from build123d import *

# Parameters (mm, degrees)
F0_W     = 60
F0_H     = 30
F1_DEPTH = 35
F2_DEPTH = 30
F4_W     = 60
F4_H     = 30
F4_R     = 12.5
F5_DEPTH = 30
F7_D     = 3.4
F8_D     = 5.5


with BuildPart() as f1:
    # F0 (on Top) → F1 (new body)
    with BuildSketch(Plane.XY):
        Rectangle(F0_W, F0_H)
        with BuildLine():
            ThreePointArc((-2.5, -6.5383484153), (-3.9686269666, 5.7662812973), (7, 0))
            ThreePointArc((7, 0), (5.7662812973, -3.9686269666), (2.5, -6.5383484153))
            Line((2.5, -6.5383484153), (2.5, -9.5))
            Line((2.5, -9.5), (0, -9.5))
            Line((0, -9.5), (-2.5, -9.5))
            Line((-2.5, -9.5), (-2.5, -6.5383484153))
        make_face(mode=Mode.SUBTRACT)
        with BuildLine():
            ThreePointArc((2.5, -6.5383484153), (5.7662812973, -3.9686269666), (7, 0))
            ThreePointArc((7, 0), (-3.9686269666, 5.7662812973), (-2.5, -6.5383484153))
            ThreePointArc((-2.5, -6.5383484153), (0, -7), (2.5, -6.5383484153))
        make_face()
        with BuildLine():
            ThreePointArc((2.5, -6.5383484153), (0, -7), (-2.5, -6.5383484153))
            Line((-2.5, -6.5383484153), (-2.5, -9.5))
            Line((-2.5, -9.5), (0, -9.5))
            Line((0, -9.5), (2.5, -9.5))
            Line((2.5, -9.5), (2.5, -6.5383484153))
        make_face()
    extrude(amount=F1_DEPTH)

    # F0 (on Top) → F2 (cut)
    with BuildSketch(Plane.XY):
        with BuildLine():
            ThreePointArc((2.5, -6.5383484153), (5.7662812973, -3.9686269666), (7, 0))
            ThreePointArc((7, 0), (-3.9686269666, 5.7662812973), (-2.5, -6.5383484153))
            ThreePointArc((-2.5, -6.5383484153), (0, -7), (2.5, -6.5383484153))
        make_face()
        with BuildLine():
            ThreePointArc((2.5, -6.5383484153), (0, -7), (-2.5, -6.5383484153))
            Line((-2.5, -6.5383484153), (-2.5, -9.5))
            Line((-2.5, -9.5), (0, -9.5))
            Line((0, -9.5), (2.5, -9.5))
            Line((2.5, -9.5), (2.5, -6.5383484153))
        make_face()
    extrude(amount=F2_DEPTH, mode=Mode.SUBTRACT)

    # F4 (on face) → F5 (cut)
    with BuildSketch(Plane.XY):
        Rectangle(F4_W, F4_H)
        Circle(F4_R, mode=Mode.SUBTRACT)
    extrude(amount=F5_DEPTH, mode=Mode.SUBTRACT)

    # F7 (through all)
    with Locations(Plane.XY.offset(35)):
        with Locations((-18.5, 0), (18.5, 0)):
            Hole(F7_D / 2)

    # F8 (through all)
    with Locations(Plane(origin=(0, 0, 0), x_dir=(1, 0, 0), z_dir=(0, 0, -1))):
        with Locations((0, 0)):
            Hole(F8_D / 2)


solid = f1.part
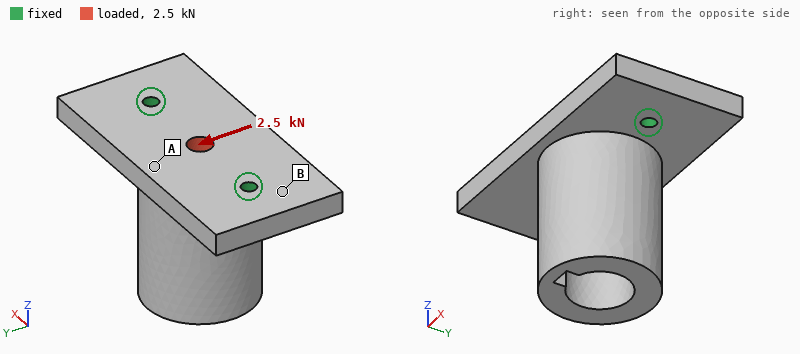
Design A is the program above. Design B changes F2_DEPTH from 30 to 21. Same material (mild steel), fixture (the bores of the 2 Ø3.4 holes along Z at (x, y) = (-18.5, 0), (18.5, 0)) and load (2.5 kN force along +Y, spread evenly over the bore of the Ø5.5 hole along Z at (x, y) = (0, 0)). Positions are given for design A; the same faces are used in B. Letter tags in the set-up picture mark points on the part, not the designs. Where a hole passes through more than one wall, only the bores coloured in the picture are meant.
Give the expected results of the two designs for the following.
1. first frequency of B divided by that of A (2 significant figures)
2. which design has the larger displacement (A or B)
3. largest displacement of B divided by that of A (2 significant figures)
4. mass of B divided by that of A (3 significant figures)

1.00
B
7.7
1.07
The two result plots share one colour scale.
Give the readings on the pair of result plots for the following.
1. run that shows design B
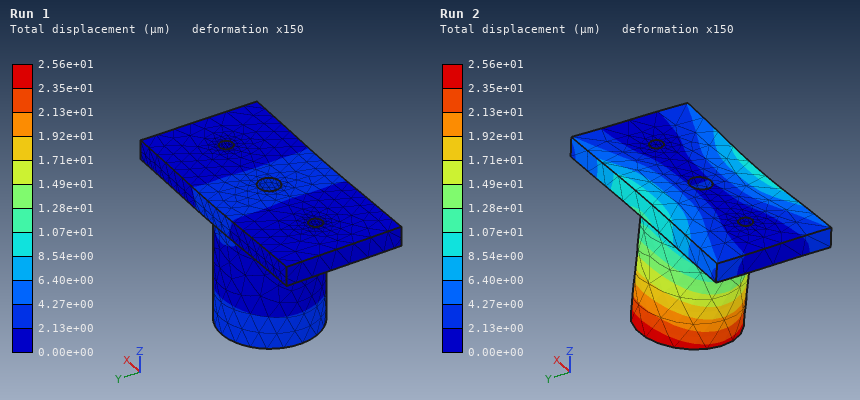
Run 2
